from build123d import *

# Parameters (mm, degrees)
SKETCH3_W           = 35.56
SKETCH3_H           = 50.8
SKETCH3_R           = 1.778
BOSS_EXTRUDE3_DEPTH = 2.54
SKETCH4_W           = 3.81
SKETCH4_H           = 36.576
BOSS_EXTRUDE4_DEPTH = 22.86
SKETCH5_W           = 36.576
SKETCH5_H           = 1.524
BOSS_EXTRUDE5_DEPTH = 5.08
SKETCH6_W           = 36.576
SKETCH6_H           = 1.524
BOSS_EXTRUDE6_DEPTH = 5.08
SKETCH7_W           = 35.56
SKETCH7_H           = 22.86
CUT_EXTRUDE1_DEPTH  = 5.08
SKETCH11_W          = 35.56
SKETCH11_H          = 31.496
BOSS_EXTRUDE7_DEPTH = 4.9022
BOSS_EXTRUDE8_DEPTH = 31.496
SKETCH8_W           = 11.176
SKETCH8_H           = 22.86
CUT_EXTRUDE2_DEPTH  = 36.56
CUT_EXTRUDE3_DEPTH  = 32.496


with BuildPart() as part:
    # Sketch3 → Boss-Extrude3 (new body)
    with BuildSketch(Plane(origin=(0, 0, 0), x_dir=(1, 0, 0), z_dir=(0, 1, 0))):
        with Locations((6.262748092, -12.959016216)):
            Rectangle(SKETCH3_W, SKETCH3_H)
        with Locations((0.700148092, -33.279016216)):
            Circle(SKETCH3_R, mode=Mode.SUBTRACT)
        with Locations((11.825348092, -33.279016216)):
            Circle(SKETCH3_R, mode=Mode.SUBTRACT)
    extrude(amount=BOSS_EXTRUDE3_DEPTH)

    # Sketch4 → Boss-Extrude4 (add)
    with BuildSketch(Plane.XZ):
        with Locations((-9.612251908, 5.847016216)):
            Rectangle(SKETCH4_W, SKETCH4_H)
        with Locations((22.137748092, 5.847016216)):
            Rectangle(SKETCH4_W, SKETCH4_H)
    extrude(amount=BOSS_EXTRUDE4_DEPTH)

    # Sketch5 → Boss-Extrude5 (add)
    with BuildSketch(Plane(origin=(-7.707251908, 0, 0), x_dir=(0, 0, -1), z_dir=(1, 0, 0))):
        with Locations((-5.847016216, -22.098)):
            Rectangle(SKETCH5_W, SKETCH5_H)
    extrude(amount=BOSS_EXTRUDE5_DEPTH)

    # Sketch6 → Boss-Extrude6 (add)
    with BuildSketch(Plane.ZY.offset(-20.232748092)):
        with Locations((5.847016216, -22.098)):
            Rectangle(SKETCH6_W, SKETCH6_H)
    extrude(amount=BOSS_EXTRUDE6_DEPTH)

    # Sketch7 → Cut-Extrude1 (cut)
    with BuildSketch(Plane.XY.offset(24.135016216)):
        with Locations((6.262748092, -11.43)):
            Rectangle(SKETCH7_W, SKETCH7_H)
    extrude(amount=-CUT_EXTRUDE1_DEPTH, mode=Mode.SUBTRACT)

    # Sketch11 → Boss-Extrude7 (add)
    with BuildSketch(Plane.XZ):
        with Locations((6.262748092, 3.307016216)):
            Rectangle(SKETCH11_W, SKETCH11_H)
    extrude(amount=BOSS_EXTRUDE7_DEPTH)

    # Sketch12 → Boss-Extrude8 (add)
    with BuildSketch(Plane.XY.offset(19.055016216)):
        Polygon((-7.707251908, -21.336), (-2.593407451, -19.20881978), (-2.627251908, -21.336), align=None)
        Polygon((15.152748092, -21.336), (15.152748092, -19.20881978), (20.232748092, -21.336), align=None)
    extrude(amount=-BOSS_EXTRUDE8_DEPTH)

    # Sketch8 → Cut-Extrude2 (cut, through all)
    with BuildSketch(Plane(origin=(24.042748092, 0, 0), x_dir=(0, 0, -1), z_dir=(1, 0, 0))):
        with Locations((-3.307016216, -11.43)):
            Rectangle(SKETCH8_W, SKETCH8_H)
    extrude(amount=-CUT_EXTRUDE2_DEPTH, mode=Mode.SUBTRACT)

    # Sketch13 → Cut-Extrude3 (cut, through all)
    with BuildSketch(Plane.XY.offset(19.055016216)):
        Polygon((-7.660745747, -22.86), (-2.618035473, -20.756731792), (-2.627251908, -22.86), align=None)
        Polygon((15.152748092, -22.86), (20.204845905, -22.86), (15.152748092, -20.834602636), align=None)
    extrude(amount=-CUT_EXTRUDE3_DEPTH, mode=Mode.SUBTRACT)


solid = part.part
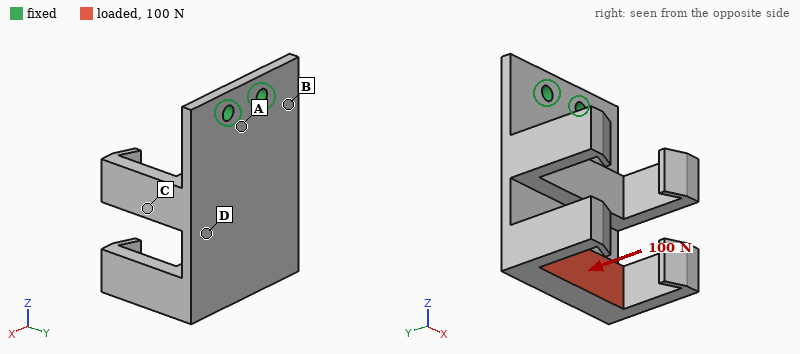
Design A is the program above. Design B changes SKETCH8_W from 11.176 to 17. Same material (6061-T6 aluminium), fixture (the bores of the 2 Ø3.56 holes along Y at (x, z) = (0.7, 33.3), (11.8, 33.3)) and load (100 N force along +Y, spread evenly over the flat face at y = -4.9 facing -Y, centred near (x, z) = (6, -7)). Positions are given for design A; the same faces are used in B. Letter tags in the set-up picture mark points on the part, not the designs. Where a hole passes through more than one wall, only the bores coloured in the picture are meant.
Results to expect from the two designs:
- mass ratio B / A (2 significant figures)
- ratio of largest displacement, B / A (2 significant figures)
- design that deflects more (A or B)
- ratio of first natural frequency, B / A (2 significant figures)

0.83
1.1
B
1.1
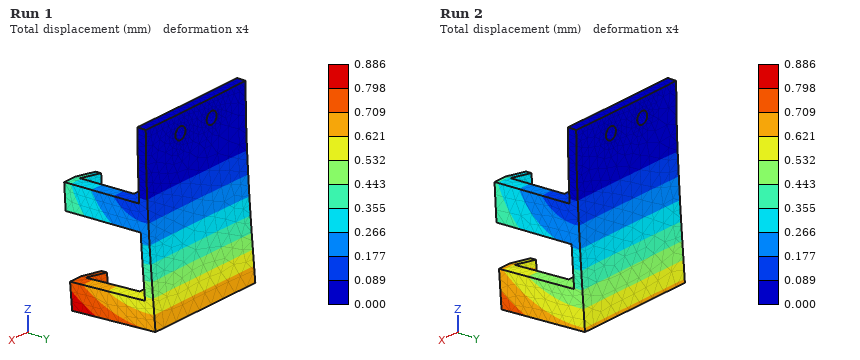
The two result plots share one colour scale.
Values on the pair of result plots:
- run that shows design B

Run 1
